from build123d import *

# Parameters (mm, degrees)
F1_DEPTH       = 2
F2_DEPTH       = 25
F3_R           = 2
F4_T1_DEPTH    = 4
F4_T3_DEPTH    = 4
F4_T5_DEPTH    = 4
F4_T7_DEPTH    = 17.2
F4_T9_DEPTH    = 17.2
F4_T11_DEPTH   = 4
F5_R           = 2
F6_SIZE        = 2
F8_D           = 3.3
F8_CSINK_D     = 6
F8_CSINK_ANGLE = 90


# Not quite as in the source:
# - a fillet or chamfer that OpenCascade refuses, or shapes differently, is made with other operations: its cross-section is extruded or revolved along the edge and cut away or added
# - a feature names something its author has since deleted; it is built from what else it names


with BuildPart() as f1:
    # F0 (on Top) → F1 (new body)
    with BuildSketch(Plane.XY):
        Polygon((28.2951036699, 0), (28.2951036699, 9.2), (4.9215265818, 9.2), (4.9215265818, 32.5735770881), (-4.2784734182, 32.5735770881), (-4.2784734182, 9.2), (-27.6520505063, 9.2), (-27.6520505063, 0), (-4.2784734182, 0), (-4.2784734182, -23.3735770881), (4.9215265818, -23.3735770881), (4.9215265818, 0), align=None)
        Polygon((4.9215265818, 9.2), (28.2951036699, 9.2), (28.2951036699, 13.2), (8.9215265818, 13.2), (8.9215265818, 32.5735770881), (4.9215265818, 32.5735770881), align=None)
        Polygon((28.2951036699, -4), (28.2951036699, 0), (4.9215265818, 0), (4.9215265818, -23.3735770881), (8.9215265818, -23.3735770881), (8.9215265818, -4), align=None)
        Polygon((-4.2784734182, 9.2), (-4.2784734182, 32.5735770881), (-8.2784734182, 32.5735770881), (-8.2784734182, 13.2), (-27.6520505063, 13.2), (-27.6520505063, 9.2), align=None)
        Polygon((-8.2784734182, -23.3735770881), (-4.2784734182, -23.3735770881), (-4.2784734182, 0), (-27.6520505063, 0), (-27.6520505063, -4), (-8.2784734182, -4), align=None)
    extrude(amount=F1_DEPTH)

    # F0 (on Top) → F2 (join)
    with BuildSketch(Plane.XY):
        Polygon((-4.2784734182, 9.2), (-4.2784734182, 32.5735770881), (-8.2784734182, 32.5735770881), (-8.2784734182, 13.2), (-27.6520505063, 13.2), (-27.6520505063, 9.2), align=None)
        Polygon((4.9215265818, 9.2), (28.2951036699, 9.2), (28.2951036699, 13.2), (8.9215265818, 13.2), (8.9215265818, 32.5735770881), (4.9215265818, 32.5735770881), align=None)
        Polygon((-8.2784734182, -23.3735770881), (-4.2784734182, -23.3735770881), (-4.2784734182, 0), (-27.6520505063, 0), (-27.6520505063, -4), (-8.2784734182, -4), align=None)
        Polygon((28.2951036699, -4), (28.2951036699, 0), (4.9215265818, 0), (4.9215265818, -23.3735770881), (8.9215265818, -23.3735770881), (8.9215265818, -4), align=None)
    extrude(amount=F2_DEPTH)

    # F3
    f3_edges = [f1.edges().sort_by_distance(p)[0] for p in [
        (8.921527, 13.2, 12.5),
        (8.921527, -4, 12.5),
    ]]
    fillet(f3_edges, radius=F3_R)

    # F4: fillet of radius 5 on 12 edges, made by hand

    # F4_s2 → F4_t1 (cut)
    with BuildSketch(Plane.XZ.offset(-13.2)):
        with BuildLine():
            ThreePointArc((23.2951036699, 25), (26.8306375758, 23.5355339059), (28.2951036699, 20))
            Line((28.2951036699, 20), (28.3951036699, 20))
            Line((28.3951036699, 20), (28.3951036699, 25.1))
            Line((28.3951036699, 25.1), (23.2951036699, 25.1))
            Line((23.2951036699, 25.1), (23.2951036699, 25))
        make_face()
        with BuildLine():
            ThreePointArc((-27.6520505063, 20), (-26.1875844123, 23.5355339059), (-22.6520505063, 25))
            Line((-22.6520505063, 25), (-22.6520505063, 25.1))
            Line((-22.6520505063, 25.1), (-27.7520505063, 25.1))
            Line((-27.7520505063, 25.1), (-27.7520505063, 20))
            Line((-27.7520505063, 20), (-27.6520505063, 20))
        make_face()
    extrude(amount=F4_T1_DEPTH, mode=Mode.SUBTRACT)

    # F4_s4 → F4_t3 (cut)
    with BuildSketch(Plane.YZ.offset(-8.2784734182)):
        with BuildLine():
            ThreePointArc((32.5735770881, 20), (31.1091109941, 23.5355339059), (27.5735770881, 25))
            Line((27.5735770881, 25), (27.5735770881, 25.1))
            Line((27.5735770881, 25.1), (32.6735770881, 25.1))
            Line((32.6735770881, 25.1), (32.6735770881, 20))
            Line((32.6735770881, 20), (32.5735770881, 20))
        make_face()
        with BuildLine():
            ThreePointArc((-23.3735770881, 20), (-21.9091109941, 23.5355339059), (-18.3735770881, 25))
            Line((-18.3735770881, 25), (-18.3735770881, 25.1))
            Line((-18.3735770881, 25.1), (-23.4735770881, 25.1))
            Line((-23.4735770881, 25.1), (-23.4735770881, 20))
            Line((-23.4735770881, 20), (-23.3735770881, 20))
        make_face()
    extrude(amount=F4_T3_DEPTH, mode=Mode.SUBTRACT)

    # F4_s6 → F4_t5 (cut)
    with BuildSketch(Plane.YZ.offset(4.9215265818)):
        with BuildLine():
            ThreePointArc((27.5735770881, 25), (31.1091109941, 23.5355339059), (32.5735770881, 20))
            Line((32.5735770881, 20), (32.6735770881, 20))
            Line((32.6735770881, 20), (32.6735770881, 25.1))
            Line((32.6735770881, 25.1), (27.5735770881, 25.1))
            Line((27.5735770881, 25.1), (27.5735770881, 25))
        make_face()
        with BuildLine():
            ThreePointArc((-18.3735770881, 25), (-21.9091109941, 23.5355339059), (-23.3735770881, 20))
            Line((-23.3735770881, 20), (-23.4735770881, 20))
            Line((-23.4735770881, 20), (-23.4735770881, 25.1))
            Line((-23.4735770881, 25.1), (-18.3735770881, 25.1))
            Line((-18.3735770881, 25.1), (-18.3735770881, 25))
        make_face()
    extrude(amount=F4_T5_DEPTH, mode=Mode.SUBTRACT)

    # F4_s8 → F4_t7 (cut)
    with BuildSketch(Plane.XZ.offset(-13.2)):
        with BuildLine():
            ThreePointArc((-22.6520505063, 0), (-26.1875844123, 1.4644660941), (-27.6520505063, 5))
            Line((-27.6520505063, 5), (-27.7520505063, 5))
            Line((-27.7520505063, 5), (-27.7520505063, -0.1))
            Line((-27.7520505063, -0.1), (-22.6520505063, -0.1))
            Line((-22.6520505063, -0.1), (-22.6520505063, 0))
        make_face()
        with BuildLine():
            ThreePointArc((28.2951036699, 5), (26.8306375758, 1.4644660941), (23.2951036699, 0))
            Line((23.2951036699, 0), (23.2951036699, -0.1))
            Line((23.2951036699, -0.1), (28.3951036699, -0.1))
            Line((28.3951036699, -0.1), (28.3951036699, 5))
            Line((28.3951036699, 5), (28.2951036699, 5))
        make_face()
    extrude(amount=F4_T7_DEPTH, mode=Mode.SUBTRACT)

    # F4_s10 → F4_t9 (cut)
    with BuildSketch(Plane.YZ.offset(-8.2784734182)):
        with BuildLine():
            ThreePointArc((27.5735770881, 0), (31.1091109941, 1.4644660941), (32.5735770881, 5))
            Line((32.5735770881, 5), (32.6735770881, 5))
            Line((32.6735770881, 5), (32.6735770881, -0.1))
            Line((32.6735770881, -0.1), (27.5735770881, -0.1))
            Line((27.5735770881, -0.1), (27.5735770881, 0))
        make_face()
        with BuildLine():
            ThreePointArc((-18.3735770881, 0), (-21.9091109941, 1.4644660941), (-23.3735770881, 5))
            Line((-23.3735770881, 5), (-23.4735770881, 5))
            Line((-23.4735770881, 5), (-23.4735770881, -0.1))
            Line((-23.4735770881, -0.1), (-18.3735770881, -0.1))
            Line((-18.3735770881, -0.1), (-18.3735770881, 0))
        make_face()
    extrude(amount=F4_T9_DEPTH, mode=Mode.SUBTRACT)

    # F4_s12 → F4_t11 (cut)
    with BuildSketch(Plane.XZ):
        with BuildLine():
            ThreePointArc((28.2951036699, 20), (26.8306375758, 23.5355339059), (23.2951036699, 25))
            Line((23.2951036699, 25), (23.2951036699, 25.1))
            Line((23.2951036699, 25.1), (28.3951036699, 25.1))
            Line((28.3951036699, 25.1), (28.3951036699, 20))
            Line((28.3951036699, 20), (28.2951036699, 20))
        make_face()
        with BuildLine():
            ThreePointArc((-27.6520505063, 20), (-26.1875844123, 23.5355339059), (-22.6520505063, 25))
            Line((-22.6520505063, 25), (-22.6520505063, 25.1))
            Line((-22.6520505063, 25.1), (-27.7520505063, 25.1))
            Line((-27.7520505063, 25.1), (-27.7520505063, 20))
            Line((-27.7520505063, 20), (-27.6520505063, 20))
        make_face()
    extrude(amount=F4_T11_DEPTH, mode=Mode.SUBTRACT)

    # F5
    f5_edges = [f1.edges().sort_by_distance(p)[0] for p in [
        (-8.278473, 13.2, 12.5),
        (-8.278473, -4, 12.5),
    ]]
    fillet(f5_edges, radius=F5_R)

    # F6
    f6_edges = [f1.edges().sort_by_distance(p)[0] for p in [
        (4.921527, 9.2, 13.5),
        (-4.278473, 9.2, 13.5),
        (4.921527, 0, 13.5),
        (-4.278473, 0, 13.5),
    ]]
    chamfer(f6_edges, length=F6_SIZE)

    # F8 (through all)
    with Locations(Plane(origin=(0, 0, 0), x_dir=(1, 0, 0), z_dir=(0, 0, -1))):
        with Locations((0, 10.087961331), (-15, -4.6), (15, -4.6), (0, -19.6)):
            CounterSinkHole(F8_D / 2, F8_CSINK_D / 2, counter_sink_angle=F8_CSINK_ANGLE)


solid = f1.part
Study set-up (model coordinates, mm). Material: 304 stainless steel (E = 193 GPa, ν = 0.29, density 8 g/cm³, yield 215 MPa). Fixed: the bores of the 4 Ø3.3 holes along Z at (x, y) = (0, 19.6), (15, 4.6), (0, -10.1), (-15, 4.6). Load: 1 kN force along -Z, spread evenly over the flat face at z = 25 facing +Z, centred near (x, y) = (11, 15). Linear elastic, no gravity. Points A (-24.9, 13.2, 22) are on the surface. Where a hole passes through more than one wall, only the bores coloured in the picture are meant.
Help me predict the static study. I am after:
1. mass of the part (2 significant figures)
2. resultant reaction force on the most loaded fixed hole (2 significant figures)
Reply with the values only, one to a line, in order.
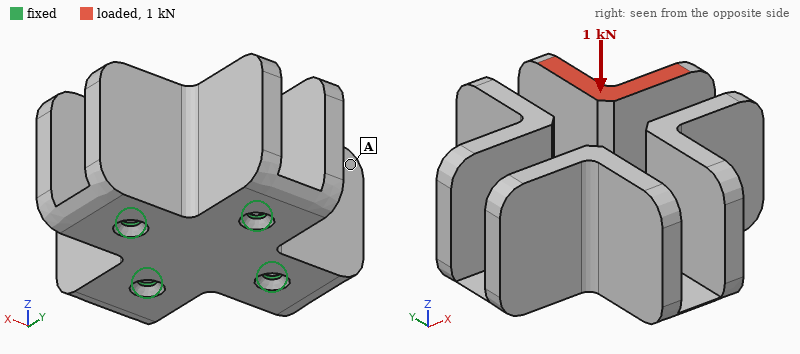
150 g
600 N
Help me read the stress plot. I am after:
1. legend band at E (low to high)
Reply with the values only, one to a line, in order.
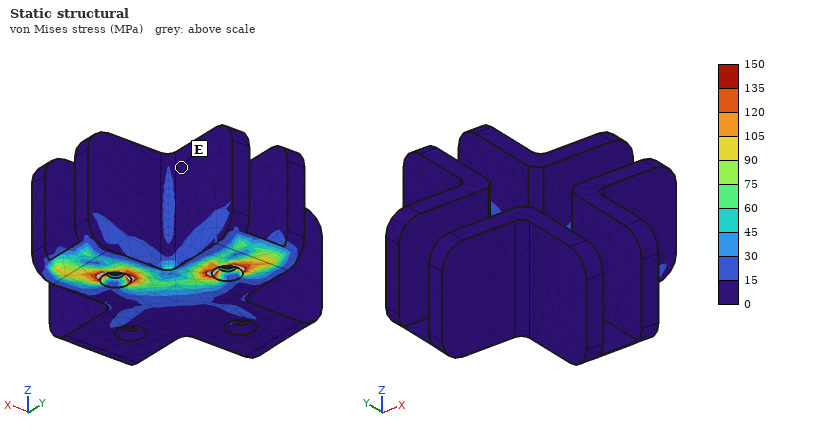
0 to 15 MPa
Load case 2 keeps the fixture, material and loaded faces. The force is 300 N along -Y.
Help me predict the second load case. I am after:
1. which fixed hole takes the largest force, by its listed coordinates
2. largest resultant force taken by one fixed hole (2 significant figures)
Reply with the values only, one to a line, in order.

(0, 19.6)
510 N
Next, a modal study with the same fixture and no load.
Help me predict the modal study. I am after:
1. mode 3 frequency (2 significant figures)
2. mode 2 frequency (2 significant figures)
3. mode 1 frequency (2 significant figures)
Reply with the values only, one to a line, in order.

2400 Hz
2400 Hz
1800 Hz
